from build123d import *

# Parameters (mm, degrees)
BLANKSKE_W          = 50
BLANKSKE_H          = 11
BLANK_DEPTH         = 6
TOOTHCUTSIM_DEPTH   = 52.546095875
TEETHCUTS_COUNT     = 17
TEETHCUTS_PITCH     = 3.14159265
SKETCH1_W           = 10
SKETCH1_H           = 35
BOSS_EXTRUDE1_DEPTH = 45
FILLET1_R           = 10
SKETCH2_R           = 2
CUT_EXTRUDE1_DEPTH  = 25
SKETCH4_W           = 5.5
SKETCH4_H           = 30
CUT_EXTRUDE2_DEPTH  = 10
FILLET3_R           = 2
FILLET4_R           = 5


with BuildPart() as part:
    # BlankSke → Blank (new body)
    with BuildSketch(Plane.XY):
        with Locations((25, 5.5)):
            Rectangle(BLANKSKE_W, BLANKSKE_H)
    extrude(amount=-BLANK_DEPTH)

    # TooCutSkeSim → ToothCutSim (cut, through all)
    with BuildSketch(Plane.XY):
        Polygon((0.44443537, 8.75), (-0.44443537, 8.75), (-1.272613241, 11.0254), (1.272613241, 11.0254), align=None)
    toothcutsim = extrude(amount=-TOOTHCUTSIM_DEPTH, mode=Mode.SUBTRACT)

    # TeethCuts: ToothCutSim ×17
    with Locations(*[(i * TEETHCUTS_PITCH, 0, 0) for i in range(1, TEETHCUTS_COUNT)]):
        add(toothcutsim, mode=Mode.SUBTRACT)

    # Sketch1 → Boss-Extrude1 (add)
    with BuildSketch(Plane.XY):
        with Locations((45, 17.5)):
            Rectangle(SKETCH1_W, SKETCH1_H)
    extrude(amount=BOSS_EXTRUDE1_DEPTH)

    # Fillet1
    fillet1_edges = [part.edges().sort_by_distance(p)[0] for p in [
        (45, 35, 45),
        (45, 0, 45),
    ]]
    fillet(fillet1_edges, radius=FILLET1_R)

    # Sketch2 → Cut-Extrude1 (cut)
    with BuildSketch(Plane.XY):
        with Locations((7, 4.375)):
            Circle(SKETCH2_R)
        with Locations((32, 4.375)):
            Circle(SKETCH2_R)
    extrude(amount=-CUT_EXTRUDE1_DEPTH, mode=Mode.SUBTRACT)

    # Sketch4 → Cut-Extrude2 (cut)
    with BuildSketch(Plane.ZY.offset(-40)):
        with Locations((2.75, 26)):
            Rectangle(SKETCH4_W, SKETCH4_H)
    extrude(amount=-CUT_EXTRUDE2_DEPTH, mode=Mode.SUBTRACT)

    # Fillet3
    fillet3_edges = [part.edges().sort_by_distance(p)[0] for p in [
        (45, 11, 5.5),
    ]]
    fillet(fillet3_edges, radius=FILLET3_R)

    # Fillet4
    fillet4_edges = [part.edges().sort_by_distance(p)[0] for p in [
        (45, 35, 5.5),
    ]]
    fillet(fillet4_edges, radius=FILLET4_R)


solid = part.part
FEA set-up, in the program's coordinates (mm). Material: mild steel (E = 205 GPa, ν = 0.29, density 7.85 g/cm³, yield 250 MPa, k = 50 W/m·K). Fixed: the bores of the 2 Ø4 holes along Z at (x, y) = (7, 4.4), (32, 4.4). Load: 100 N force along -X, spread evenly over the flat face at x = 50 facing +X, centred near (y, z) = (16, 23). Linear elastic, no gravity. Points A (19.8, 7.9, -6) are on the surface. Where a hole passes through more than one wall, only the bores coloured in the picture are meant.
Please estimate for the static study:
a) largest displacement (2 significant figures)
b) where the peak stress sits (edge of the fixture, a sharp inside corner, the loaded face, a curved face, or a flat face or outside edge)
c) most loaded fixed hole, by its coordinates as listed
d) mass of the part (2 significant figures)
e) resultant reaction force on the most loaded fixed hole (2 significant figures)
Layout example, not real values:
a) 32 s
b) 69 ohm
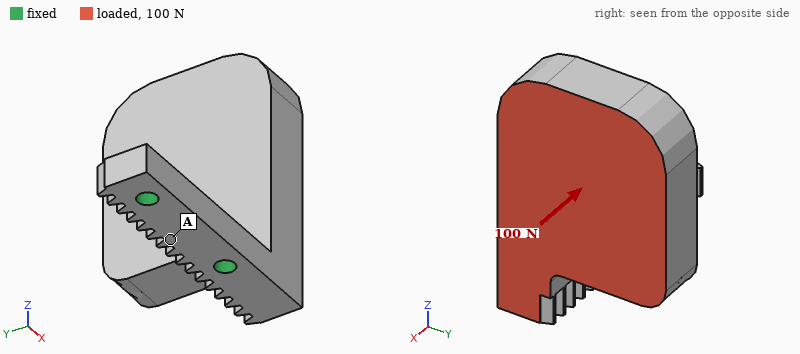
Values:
a) 50 µm
b) a flat face or outside edge
c) (32, 4.4)
d) 130 g
e) 97 N
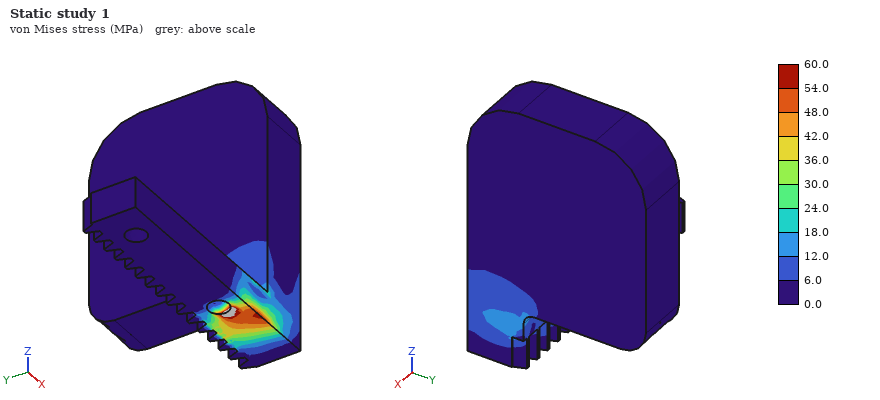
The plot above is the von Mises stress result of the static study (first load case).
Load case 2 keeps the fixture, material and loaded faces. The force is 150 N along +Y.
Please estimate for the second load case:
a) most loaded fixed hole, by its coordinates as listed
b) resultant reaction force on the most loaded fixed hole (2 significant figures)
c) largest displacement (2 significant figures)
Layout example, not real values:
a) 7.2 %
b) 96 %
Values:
a) (32, 4.4)
b) 170 N
c) 67 µm
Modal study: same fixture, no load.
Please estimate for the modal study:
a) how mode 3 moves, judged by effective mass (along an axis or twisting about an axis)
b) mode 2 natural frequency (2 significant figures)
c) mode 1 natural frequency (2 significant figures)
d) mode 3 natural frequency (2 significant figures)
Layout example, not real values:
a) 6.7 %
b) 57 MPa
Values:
a) twisting about Z
b) 840 Hz
c) 800 Hz
d) 2700 Hz
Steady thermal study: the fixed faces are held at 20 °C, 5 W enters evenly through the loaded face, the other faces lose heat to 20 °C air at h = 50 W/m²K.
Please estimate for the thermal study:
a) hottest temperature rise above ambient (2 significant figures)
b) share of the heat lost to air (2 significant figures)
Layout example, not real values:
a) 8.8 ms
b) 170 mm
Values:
a) 18 K
b) 49 %
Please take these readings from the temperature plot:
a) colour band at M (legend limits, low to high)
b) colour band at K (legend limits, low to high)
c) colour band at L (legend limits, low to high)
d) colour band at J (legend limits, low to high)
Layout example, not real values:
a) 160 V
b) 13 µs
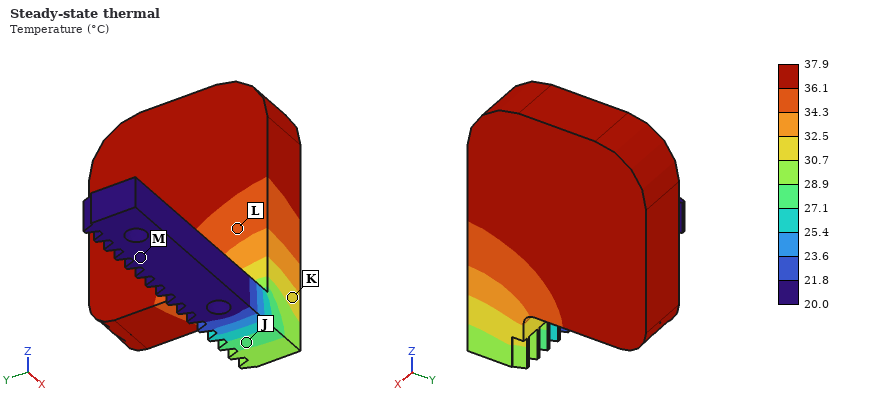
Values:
a) 20.0 to 21.8 °C
b) 30.7 to 32.5 °C
c) 34.3 to 36.1 °C
d) 27.1 to 28.9 °C
